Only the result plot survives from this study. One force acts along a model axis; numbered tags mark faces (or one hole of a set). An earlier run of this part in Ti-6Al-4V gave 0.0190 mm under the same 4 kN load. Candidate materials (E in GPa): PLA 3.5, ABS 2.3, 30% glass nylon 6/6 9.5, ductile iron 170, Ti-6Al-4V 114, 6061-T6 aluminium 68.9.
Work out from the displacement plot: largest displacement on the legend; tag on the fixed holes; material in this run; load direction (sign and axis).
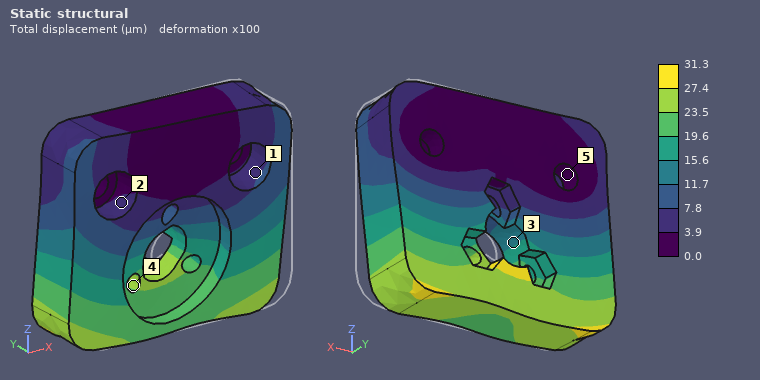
31.3 µm
5
6061-T6 aluminium
-X
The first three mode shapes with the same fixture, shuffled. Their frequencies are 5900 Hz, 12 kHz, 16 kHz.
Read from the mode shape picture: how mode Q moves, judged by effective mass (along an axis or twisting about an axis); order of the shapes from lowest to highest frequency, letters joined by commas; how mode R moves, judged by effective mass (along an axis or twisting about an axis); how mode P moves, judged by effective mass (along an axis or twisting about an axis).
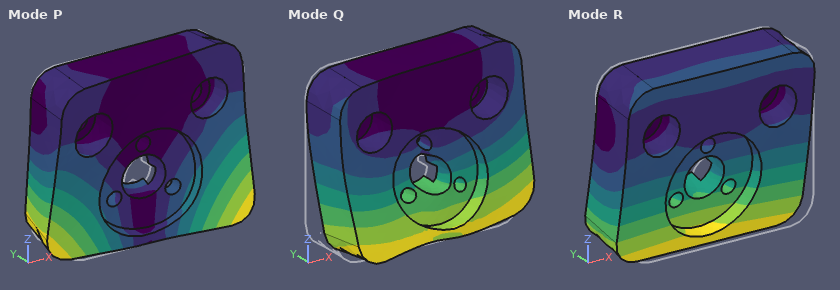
along X
R, P, Q
along Y
twisting about Z
